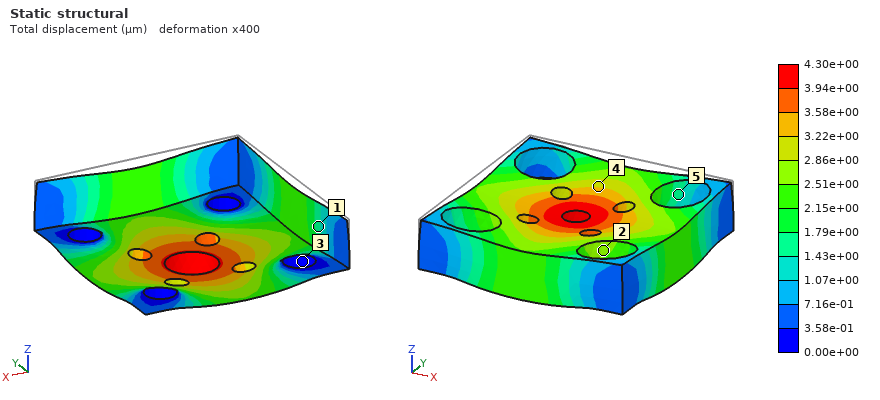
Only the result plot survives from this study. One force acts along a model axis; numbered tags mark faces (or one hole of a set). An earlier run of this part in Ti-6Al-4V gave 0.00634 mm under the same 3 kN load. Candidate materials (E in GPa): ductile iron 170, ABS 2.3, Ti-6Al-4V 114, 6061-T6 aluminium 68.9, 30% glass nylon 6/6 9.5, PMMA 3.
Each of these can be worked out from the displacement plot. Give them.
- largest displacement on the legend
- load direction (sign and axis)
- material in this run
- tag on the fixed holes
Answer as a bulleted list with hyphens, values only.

- 4.30e+00 µm
- -Z
- ductile iron
- 3
